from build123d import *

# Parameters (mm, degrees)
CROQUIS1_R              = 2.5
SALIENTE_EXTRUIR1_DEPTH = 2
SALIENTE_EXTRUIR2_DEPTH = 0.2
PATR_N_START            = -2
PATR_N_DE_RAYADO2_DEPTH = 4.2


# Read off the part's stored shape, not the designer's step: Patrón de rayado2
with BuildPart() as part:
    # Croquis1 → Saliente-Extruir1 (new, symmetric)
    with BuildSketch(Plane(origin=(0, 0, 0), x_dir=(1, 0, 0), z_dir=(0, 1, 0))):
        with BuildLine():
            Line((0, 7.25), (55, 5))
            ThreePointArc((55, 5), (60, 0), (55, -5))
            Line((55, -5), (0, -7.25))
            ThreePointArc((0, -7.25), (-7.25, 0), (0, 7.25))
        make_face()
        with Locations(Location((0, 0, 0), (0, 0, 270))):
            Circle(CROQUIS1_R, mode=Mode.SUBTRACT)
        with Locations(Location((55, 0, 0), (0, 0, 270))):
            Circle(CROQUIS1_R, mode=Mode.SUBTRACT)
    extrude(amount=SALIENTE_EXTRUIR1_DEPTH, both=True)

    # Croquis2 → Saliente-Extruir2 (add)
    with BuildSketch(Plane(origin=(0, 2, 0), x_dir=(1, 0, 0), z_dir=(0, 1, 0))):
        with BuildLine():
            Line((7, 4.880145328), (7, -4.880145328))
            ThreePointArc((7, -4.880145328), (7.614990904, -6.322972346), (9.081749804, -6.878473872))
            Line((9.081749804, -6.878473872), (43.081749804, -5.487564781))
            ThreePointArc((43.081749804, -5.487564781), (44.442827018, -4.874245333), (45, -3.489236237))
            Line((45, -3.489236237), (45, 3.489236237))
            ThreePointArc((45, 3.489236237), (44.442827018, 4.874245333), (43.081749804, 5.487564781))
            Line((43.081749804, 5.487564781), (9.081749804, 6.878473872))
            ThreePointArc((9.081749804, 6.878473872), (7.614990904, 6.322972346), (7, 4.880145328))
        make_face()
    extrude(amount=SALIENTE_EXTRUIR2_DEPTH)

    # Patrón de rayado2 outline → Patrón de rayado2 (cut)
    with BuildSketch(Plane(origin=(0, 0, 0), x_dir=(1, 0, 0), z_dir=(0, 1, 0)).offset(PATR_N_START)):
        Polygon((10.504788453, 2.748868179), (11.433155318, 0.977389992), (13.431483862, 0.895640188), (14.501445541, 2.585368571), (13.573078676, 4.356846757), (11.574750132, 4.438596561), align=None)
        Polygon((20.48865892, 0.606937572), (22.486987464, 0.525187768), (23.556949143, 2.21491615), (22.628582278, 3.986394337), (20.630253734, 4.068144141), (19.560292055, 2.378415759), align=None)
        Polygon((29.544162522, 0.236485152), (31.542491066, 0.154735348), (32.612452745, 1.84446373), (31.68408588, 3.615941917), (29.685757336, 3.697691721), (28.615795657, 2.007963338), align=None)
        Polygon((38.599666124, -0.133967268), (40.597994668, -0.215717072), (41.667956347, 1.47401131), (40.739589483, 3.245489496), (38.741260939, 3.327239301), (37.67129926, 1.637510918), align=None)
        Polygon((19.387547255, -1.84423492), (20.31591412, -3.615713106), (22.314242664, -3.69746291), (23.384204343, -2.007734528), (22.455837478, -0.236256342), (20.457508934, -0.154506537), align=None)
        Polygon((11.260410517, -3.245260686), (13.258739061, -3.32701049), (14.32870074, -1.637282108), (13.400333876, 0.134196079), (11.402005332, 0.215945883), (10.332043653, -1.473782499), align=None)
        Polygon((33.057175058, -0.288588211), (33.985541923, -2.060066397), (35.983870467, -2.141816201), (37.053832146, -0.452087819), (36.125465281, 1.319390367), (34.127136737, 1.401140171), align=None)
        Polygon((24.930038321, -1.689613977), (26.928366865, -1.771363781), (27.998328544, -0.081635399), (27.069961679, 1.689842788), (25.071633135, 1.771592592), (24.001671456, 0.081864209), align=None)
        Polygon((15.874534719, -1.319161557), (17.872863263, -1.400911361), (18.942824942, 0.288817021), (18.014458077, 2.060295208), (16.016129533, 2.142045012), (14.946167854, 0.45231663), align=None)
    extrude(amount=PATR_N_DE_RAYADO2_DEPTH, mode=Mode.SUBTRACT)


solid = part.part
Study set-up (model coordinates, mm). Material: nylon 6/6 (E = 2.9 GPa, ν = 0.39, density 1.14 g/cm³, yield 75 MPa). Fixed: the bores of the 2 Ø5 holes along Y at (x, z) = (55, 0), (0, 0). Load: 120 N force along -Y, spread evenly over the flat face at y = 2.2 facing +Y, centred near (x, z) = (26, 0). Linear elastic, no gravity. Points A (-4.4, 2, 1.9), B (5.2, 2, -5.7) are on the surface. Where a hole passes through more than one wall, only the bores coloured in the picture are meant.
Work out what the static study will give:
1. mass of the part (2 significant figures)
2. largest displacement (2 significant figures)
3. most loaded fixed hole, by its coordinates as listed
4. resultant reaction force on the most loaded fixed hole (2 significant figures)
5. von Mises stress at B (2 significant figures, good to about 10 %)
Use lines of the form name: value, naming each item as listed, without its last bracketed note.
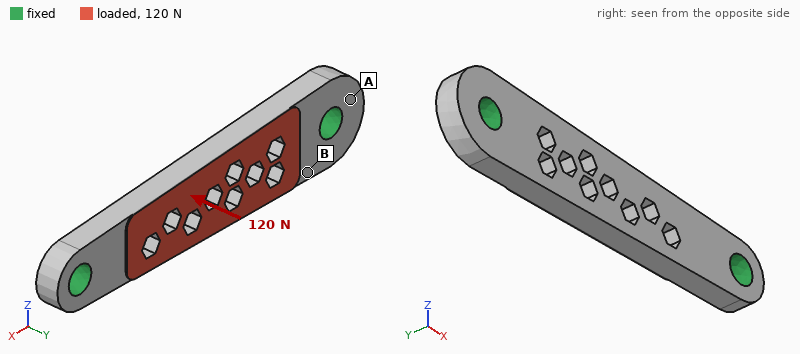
mass of the part: 3.1 g
largest displacement: 0.37 mm
most loaded fixed hole, by its coordinates as listed: (0, 0)
resultant reaction force on the most loaded fixed hole: 68 N
von Mises stress at B: 11 MPa
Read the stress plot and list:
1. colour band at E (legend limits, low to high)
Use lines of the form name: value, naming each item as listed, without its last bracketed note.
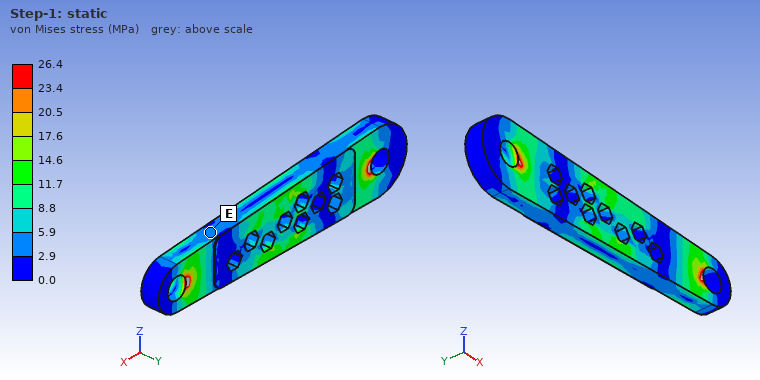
colour band at E: 2.9 to 5.9 MPa
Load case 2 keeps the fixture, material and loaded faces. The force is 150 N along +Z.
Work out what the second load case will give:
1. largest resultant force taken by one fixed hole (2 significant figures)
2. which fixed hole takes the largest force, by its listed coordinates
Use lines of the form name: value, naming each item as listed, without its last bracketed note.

largest resultant force taken by one fixed hole: 82 N
which fixed hole takes the largest force, by its listed coordinates: (0, 0)
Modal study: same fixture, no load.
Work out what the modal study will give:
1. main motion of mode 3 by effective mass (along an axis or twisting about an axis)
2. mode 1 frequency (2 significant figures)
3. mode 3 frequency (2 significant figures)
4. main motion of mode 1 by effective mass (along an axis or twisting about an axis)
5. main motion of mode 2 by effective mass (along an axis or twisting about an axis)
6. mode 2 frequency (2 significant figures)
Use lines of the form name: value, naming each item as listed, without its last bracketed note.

main motion of mode 3 by effective mass: twisting about X
mode 1 frequency: 2400 Hz
mode 3 frequency: 4900 Hz
main motion of mode 1 by effective mass: along Y
main motion of mode 2 by effective mass: along Z
mode 2 frequency: 4500 Hz
